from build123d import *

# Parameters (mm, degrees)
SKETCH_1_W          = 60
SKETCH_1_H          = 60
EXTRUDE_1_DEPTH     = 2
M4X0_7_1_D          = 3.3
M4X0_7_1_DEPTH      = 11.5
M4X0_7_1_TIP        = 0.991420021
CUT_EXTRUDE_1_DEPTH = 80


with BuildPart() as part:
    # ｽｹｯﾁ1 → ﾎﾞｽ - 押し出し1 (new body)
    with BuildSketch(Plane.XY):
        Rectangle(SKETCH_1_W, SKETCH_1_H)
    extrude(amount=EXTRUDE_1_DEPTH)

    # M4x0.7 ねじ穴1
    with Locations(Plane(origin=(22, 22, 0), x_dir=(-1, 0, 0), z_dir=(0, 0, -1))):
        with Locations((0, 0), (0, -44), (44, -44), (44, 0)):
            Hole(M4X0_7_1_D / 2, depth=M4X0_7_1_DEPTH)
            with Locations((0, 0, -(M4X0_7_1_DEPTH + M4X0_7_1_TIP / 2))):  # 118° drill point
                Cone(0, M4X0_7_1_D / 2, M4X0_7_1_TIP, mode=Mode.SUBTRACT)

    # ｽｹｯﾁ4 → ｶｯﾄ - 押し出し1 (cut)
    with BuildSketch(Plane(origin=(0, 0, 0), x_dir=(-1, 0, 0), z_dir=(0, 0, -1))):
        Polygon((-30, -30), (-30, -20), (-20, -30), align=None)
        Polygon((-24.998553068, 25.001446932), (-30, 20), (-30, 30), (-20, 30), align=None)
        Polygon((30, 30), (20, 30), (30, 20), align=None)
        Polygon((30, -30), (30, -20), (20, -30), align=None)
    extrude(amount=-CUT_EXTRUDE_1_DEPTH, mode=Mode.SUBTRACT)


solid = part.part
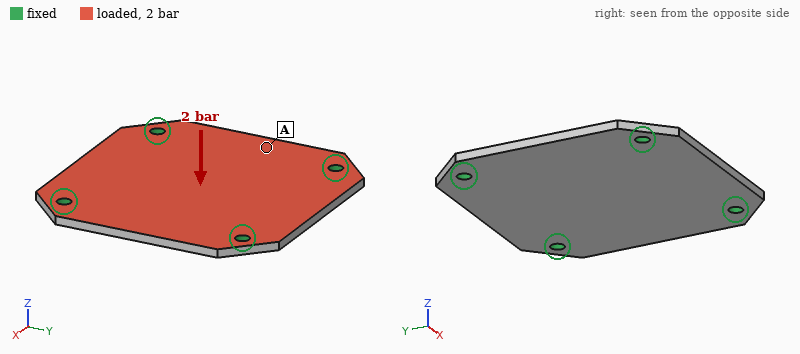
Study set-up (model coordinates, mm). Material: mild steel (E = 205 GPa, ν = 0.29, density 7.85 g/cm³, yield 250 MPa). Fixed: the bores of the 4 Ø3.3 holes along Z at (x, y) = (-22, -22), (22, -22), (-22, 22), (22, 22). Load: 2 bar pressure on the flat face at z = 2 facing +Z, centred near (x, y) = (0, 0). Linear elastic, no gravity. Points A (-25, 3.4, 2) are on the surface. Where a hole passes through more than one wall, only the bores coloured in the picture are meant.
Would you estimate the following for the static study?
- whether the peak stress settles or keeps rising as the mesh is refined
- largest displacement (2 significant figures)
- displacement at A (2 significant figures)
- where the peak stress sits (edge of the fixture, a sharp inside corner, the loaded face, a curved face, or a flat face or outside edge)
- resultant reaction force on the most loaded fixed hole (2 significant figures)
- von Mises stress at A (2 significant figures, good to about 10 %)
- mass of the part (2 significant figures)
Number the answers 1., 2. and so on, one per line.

1. keeps rising
2. 33 µm
3. 15 µm
4. edge of the fixture
5. 170 N
6. 26 MPa
7. 53 g
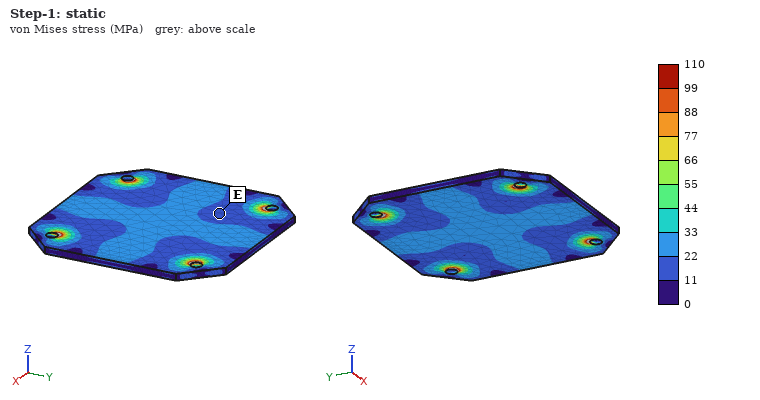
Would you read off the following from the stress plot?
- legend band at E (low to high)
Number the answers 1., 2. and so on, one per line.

1. 11 to 22 MPa
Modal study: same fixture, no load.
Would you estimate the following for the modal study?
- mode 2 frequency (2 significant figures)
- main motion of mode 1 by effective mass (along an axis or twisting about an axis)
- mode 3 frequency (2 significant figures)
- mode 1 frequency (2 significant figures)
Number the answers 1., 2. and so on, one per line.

1. 5900 Hz
2. along Z
3. 5900 Hz
4. 3800 Hz
